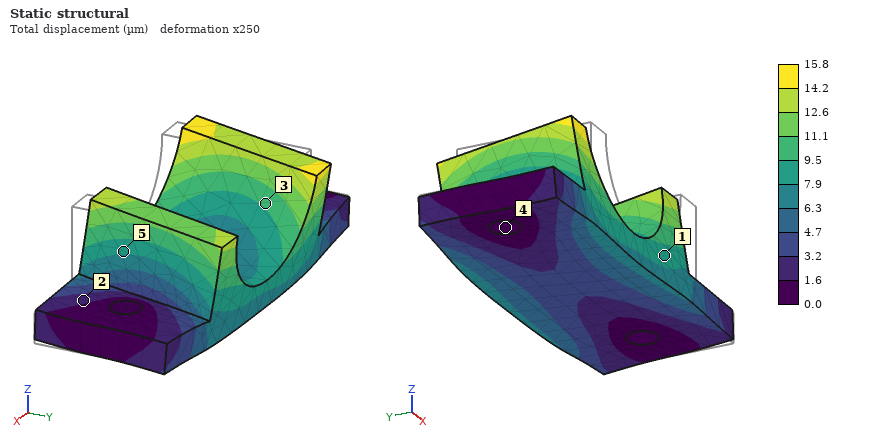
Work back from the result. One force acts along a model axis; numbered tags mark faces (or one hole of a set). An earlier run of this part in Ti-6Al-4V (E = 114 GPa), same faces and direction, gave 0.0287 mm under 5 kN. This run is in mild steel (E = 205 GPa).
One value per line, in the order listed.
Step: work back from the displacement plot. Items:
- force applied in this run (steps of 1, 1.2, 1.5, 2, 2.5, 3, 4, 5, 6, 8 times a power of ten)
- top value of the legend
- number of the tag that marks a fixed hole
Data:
5 kN
15.8 µm
4
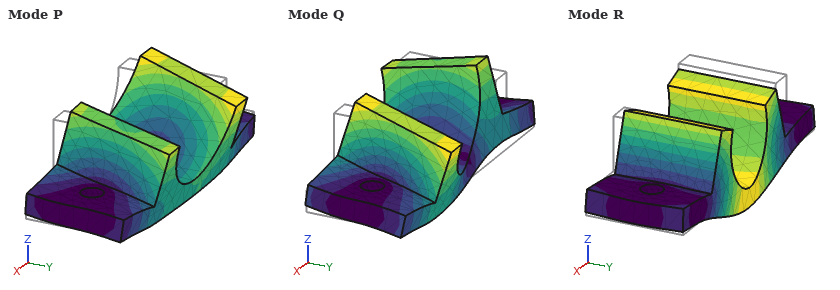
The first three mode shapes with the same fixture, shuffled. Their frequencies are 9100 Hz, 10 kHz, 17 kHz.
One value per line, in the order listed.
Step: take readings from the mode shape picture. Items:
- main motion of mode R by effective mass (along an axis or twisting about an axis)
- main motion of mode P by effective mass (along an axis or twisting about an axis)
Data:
along Z
along Y
